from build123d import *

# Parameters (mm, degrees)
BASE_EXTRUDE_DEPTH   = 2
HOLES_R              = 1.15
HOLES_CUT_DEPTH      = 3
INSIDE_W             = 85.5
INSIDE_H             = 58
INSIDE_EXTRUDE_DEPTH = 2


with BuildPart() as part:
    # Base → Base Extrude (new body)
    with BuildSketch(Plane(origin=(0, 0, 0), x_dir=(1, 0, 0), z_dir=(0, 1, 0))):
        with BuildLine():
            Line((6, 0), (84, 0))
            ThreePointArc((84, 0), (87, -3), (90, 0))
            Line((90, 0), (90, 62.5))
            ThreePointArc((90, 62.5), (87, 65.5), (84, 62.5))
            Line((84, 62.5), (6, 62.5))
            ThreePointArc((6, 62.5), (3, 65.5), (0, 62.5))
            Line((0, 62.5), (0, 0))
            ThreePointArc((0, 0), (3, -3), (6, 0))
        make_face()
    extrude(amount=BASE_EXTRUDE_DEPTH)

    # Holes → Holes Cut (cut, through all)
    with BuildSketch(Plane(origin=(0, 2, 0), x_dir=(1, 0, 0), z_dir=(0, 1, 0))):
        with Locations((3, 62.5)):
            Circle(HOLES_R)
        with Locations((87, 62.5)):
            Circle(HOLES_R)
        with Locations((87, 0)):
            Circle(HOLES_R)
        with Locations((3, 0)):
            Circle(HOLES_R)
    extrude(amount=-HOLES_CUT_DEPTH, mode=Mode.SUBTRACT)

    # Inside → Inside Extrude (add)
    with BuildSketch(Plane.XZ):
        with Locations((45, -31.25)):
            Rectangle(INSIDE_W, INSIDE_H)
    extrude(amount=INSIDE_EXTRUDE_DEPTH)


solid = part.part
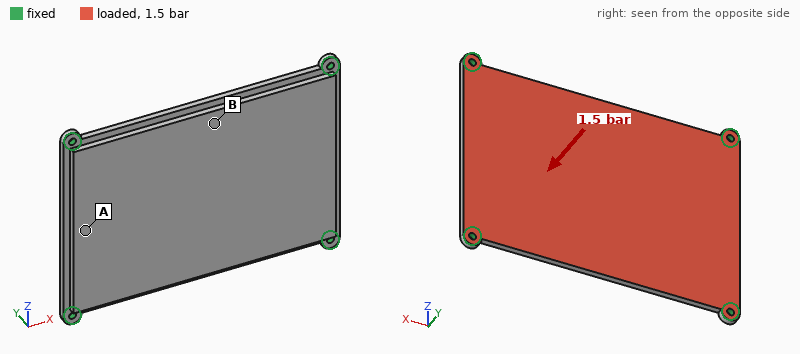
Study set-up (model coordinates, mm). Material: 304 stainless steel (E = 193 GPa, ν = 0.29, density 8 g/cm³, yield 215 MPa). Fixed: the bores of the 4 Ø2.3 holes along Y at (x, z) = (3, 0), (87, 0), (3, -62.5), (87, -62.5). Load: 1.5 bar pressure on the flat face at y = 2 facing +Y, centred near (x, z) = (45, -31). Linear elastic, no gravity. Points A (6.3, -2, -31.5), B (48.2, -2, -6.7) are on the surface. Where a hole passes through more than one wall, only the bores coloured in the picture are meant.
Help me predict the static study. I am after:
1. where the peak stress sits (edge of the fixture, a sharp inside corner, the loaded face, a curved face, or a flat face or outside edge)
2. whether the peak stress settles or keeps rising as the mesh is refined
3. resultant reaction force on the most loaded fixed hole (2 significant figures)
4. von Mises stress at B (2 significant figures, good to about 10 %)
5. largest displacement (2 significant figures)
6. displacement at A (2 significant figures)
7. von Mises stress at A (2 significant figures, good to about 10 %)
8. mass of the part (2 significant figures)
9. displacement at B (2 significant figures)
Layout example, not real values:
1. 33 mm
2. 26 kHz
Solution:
1. edge of the fixture
2. keeps rising
3. 550 N
4. 39 MPa
5. 70 µm
6. 28 µm
7. 27 MPa
8. 170 g
9. 66 µm
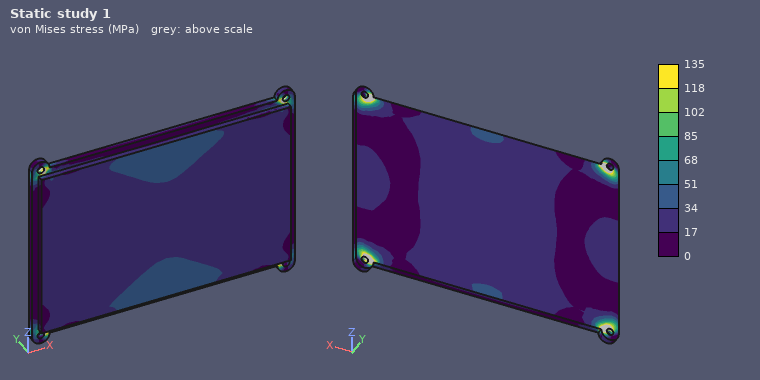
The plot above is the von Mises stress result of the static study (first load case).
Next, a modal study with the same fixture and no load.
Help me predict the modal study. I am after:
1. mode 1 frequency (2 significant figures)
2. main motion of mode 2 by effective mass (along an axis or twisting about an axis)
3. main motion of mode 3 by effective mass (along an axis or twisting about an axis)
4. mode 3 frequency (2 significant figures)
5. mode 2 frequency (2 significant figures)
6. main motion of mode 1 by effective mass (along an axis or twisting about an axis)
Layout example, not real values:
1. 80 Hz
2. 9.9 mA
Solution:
1. 1500 Hz
2. twisting about X
3. twisting about Z
4. 3500 Hz
5. 3000 Hz
6. along Y
